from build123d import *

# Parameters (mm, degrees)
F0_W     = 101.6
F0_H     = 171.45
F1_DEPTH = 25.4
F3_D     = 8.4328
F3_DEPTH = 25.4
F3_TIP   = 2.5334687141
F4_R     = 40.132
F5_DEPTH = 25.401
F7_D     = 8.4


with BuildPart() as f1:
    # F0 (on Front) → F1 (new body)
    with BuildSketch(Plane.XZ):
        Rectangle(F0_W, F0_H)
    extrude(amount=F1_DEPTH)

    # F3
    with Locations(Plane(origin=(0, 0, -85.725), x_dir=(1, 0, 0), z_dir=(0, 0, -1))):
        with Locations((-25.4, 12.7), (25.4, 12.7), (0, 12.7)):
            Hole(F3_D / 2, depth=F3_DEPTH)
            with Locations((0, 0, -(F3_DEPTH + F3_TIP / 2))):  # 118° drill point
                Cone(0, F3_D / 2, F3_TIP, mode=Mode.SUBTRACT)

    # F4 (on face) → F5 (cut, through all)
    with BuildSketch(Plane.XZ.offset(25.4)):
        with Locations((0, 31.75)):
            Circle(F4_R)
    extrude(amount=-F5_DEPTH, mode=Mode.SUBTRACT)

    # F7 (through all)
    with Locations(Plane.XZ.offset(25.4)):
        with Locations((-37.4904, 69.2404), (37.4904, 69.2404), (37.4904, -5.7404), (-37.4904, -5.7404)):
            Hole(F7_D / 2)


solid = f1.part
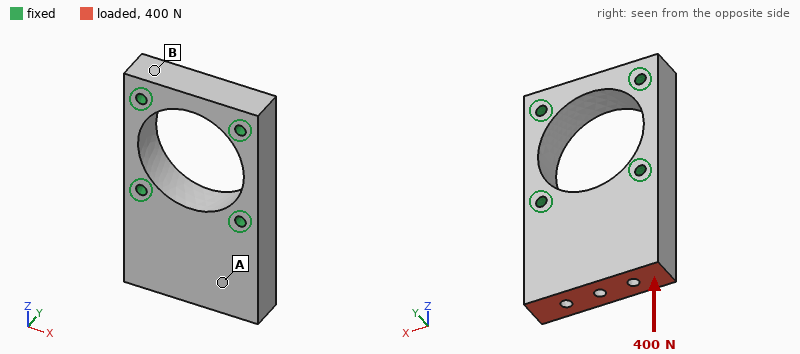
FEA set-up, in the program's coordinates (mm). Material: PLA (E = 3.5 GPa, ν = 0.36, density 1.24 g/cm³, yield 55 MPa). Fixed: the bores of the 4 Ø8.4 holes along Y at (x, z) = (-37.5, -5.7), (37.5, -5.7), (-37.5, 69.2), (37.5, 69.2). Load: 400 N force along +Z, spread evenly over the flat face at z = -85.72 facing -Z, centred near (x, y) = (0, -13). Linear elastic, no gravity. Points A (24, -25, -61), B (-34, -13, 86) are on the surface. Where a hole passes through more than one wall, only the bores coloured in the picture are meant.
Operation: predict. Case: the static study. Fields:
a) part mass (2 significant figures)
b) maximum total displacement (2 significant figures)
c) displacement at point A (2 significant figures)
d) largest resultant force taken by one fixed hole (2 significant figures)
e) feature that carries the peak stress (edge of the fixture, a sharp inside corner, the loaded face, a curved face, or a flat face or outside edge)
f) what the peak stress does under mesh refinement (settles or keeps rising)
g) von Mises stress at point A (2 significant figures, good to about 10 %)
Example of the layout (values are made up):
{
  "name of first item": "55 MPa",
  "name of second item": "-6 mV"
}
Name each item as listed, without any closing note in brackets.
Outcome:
{
  "part mass": "380 g",
  "maximum total displacement": "4.7 µm",
  "displacement at point A": "3.5 µm",
  "largest resultant force taken by one fixed hole": "200 N",
  "feature that carries the peak stress": "edge of the fixture",
  "what the peak stress does under mesh refinement": "keeps rising",
  "von Mises stress at point A": "0.16 MPa"
}
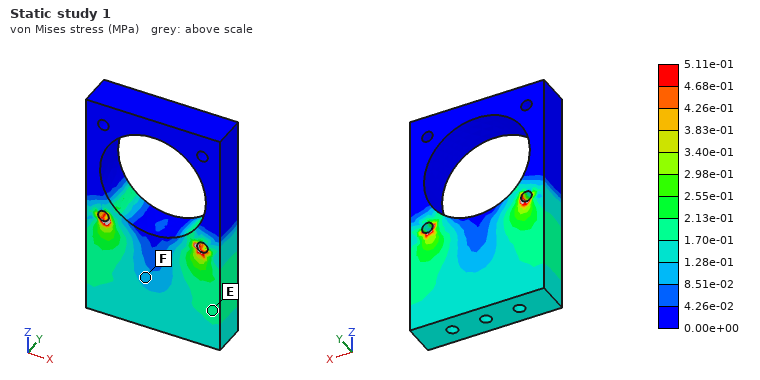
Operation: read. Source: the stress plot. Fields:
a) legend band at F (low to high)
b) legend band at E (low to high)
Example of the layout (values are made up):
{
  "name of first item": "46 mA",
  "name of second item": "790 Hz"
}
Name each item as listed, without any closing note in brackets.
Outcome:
{
  "legend band at F": "8.51e-02 to 1.28e-01 MPa",
  "legend band at E": "1.70e-01 to 2.13e-01 MPa"
}
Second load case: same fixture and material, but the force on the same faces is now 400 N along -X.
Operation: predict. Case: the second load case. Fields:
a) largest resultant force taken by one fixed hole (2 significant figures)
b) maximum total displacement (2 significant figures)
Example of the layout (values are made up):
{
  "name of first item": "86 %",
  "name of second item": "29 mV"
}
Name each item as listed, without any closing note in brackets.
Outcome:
{
  "largest resultant force taken by one fixed hole": "430 N",
  "maximum total displacement": "27 µm"
}
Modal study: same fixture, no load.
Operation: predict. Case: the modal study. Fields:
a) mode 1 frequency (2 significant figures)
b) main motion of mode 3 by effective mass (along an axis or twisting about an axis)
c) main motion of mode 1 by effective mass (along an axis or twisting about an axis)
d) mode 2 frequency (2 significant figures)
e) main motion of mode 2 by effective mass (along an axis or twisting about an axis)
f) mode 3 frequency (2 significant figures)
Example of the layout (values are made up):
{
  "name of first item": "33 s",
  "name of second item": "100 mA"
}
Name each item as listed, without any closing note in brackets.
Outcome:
{
  "mode 1 frequency": "820 Hz",
  "main motion of mode 3 by effective mass": "along X",
  "main motion of mode 1 by effective mass": "along Y",
  "mode 2 frequency": "1800 Hz",
  "main motion of mode 2 by effective mass": "twisting about Z",
  "mode 3 frequency": "2300 Hz"
}
